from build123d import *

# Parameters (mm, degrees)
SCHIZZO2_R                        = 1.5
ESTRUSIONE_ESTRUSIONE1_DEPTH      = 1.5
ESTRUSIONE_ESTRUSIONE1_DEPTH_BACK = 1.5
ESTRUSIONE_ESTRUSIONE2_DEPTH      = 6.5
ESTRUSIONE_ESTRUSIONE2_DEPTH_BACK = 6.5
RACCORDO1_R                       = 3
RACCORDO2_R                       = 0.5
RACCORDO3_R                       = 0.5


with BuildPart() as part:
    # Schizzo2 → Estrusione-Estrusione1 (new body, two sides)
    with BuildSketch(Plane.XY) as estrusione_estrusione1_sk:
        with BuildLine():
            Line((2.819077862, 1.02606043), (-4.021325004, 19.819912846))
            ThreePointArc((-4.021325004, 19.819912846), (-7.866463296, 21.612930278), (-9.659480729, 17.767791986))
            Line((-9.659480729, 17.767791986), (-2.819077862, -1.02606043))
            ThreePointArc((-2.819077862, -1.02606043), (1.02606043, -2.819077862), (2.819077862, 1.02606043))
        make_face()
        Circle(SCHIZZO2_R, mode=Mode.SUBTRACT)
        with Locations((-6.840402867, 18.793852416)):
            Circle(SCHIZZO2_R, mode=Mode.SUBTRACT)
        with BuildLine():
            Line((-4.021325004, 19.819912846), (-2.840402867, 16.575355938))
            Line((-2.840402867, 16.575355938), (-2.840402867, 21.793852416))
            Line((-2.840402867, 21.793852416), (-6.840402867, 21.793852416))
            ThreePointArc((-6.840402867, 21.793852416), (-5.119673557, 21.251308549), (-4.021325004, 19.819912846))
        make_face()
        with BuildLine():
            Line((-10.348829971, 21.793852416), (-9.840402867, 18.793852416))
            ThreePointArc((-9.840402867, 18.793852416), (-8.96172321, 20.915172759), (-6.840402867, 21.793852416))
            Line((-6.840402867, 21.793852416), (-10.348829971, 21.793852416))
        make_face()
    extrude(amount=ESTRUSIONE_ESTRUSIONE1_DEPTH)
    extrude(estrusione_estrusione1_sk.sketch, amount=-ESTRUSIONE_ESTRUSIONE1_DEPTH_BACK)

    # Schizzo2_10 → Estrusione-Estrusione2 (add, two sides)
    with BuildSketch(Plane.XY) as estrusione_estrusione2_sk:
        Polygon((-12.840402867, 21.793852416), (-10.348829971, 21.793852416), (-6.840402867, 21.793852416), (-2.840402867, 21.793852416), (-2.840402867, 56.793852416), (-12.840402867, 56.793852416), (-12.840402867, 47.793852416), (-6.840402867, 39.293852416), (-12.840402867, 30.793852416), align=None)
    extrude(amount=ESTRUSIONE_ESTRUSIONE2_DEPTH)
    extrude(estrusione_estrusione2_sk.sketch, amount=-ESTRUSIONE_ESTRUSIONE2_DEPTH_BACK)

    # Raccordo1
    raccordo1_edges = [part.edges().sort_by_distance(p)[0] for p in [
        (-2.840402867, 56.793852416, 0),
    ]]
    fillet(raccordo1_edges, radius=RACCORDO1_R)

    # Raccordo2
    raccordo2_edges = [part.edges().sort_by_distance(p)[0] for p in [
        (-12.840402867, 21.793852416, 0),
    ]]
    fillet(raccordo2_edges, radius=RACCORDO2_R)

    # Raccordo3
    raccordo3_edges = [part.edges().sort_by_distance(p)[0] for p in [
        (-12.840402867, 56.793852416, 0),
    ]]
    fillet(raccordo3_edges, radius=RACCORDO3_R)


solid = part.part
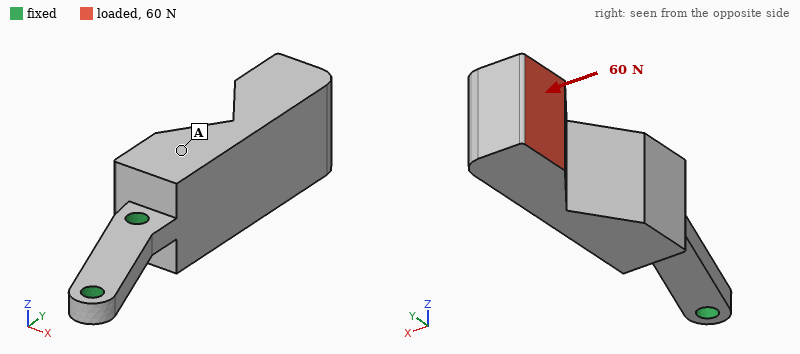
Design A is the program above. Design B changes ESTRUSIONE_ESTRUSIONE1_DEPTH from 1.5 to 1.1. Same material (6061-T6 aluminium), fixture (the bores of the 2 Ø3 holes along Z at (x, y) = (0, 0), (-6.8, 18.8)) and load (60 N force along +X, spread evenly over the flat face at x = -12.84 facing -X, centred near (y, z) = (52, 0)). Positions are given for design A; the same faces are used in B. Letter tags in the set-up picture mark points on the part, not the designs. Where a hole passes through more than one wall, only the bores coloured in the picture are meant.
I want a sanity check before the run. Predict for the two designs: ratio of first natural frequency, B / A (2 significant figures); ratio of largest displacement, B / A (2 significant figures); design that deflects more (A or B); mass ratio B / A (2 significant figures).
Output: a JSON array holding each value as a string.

["0.83", "1.1", "B", "0.99"]
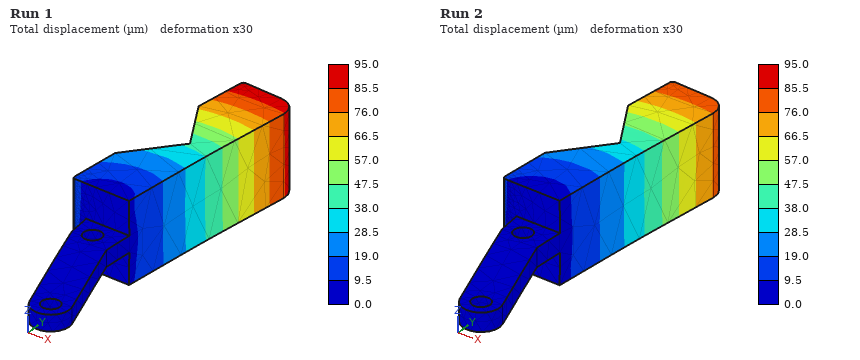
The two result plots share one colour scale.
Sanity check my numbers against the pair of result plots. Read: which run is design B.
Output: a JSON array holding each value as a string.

["Run 1"]
